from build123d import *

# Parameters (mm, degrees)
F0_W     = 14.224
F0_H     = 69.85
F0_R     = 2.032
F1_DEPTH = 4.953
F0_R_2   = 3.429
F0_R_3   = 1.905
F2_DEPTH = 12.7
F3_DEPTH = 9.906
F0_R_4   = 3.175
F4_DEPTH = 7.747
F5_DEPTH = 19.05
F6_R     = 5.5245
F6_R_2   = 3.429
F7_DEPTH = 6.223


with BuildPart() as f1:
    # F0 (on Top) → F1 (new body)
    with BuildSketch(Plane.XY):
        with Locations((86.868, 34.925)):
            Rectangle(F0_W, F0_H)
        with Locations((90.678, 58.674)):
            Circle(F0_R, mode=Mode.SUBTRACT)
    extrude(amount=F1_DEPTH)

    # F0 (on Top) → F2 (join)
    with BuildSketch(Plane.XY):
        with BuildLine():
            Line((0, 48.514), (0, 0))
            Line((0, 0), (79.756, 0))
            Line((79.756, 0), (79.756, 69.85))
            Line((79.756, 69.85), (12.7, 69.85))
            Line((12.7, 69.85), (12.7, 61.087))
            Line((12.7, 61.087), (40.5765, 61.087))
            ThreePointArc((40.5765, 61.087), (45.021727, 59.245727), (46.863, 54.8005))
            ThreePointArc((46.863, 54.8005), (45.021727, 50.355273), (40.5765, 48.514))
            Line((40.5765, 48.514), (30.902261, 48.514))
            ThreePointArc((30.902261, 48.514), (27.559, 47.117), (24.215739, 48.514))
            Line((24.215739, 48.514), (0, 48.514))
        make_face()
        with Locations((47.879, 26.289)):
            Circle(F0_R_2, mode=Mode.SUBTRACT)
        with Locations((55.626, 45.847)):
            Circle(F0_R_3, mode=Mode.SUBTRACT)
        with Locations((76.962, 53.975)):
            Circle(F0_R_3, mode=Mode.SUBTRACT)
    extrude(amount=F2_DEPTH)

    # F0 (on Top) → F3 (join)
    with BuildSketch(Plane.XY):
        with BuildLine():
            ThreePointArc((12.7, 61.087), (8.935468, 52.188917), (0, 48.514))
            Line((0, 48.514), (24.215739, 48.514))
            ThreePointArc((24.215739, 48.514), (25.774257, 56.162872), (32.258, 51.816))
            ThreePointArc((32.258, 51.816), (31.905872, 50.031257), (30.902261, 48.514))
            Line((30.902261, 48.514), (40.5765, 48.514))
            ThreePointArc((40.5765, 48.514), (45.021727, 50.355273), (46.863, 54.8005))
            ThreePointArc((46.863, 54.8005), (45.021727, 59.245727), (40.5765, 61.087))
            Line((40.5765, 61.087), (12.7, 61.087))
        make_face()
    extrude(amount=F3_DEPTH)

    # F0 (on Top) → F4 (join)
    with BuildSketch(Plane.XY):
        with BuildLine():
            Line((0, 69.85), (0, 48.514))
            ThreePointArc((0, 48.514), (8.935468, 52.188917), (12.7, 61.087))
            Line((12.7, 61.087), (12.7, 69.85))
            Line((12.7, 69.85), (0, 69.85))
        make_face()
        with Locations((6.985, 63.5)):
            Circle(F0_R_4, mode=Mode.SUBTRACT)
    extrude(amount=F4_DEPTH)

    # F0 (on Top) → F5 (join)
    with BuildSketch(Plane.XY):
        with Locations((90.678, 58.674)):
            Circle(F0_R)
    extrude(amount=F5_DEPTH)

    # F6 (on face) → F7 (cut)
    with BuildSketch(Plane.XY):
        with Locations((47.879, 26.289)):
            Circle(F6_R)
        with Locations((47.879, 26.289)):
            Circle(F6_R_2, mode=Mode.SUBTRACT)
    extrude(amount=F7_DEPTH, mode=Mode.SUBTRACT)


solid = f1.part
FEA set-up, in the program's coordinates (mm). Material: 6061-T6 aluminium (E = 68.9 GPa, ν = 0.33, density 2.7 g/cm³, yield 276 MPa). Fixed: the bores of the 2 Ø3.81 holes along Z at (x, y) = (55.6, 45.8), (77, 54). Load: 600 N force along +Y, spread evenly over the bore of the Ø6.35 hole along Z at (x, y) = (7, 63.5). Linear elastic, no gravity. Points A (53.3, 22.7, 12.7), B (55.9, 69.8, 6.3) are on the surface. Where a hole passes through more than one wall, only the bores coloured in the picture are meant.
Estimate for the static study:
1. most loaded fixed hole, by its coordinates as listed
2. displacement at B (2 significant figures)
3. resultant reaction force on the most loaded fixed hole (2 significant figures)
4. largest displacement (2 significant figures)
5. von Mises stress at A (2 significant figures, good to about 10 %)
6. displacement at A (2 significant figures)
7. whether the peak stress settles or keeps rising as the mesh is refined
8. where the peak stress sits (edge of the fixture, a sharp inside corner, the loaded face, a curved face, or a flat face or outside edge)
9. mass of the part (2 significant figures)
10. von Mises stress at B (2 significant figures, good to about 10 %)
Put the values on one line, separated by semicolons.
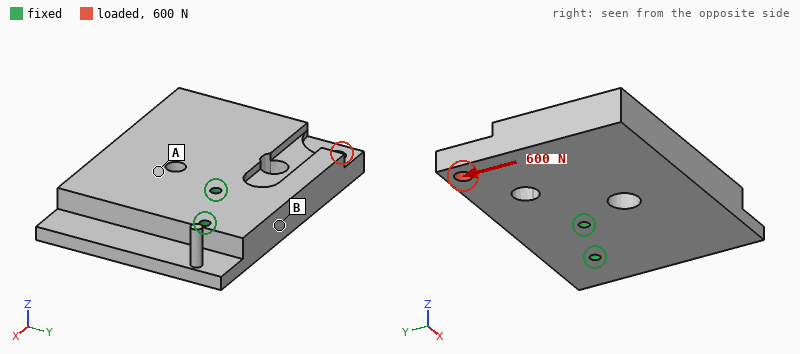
(55.6, 45.8); 2.9 µm; 1.7 kN; 15 µm; 2.8 MPa; 4.2 µm; keeps rising; edge of the fixture; 190 g; 5.6 MPa
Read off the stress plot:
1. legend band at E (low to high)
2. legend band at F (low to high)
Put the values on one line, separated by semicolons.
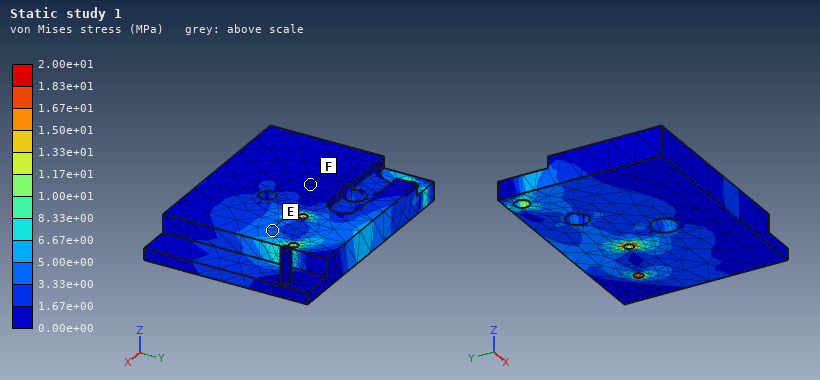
3.33e+00 to 5.00e+00 MPa; 0.00e+00 to 1.67e+00 MPa
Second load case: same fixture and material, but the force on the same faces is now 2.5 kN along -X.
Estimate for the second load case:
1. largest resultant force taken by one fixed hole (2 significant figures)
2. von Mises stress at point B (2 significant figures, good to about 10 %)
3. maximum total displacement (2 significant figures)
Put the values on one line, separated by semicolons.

1.9 kN; 11 MPa; 32 µm
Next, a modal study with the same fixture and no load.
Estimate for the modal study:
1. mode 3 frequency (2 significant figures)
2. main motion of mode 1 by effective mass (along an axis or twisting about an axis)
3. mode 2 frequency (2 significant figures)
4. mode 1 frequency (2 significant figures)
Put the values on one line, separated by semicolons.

4100 Hz; along Z; 3200 Hz; 2200 Hz
